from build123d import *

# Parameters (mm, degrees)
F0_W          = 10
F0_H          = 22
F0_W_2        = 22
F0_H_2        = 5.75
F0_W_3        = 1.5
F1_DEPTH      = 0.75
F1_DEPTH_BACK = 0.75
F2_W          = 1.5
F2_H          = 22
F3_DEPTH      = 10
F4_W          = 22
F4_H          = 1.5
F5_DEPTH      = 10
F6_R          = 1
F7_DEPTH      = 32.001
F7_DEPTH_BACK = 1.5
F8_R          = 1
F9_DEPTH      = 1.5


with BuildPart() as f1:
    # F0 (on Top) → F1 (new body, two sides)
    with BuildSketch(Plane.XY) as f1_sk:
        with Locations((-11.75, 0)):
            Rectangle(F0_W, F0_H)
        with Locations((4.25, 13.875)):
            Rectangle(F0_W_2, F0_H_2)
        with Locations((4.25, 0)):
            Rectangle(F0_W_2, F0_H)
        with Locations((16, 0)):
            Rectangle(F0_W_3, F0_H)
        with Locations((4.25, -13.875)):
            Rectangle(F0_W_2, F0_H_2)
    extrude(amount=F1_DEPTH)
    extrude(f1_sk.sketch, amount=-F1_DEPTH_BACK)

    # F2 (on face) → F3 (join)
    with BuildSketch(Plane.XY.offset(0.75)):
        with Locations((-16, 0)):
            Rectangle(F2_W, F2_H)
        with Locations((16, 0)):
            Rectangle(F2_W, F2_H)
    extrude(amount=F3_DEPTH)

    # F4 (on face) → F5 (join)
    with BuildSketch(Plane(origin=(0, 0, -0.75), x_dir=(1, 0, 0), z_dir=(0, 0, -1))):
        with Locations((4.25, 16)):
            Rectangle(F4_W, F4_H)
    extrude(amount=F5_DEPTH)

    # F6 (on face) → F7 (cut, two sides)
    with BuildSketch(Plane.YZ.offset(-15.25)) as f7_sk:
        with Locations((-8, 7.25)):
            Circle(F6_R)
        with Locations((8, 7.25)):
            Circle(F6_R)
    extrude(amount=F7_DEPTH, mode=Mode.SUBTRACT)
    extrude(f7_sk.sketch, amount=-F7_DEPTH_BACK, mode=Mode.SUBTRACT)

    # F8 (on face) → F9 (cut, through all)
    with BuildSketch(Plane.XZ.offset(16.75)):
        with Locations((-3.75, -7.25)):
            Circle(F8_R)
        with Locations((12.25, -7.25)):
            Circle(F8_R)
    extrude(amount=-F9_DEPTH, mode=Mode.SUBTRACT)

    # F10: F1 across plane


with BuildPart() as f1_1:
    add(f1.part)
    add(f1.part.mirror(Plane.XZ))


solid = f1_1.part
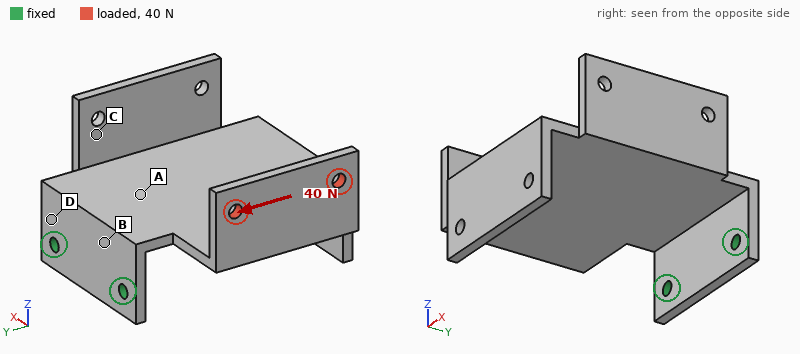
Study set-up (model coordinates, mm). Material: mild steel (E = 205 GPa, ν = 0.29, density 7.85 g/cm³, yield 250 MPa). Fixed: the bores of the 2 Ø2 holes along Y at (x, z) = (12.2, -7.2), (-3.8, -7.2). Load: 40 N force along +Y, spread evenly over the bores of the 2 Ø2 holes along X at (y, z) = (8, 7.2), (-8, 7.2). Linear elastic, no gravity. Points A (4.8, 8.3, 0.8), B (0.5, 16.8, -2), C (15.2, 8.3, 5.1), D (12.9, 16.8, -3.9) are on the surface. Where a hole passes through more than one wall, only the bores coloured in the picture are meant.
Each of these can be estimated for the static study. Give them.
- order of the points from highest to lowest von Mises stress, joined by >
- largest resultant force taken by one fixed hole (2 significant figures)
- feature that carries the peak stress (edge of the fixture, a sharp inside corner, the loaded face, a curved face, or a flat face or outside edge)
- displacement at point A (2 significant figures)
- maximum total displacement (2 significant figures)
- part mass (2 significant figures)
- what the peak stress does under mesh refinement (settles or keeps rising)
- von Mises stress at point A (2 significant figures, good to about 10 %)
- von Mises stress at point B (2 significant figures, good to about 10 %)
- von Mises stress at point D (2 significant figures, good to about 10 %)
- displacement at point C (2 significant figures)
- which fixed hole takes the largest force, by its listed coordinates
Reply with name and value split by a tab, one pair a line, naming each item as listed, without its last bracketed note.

order of the points from highest to lowest von Mises stress, joined by >	B > D > A > C
largest resultant force taken by one fixed hole	69 N
feature that carries the peak stress	edge of the fixture
displacement at point A	0.028 mm
maximum total displacement	0.18 mm
part mass	22 g
what the peak stress does under mesh refinement	keeps rising
von Mises stress at point A	21 MPa
von Mises stress at point B	54 MPa
von Mises stress at point D	40 MPa
displacement at point C	0.028 mm
which fixed hole takes the largest force, by its listed coordinates	(-3.8, -7.2)
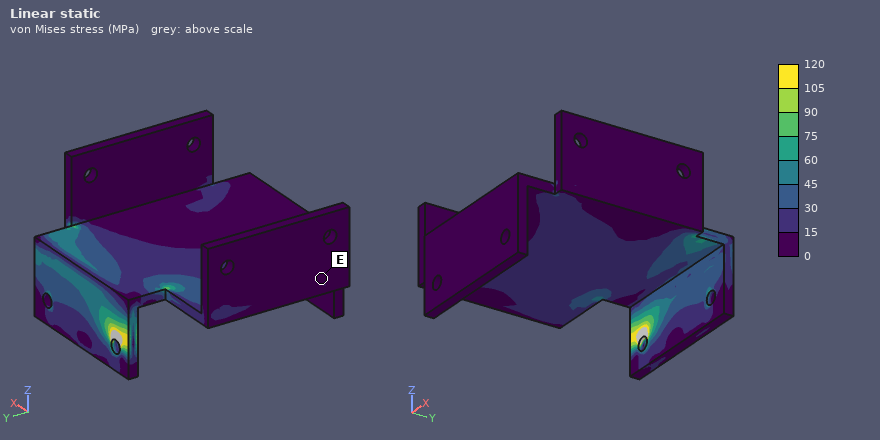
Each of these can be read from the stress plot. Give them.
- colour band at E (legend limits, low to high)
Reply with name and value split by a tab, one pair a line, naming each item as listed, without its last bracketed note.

colour band at E	0 to 15 MPa
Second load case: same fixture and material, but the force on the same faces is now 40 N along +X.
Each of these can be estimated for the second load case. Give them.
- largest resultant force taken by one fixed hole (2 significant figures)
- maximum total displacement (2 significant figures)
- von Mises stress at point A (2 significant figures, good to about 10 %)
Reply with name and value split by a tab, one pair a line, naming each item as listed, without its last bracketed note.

largest resultant force taken by one fixed hole	57 N
maximum total displacement	74 µm
von Mises stress at point A	14 MPa
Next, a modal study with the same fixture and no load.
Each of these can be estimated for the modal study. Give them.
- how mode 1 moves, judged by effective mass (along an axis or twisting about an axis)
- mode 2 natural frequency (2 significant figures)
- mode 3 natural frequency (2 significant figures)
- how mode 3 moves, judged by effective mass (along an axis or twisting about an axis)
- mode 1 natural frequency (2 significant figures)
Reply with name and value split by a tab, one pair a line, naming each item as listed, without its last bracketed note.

how mode 1 moves, judged by effective mass	along Z
mode 2 natural frequency	1200 Hz
mode 3 natural frequency	1800 Hz
how mode 3 moves, judged by effective mass	along X
mode 1 natural frequency	540 Hz
